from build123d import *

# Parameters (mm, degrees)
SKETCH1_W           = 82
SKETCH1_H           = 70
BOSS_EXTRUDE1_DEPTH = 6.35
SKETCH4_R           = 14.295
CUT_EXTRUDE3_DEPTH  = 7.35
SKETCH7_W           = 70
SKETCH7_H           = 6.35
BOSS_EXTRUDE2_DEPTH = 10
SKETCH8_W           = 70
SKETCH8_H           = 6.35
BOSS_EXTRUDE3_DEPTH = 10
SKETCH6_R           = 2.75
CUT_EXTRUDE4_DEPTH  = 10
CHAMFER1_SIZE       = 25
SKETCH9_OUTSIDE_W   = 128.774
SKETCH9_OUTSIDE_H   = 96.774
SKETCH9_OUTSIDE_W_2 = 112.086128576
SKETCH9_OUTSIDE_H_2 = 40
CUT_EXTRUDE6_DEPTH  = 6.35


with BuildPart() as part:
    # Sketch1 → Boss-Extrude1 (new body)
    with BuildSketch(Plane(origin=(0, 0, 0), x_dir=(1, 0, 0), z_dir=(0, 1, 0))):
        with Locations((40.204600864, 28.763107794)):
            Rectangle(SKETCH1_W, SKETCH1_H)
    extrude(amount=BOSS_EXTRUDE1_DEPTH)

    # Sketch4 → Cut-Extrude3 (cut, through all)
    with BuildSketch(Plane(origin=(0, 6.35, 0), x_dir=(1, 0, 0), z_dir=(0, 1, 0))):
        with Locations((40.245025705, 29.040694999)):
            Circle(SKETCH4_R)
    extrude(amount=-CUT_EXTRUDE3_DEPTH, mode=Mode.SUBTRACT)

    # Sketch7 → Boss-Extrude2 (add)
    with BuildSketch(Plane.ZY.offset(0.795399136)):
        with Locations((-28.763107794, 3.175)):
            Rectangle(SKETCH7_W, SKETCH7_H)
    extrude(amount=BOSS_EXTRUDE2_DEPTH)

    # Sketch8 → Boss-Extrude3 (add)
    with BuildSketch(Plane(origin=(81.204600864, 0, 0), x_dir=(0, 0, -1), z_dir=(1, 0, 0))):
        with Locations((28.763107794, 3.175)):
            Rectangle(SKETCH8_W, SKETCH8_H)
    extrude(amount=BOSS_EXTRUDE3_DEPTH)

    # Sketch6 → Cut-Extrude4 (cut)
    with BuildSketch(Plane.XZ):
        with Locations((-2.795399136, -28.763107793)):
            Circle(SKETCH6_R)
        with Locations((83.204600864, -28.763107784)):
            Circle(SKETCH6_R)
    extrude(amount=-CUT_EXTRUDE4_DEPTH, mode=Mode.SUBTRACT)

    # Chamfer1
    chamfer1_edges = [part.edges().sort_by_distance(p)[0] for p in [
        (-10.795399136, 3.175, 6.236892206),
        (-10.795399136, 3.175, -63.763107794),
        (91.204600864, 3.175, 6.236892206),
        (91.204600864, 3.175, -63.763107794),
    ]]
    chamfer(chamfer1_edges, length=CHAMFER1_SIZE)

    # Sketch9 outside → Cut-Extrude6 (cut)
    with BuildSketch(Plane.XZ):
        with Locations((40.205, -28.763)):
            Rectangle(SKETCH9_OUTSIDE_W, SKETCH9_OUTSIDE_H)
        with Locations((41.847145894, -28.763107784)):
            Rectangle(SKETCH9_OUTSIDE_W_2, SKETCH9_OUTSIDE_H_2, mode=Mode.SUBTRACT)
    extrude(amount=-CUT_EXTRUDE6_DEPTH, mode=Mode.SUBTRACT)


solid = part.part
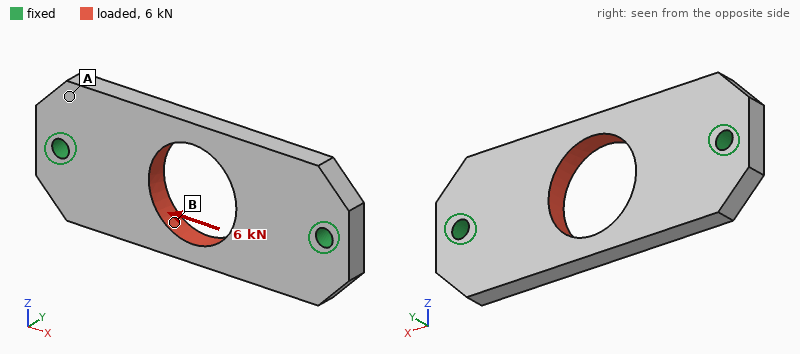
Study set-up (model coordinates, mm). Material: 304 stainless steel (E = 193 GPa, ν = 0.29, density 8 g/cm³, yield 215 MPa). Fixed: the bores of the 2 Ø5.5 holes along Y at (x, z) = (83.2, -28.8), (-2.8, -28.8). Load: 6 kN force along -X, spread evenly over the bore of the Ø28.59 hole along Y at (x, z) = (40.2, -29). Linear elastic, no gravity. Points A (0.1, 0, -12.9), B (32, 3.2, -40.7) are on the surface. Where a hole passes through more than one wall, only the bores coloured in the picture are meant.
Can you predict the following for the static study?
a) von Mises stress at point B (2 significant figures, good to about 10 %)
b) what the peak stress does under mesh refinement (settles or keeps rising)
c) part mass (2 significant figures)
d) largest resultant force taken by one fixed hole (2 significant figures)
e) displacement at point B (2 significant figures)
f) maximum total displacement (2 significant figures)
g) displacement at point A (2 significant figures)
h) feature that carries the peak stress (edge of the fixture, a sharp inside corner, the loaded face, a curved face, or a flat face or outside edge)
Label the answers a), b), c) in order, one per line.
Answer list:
a) 21 MPa
b) keeps rising
c) 160 g
d) 3.0 kN
e) 3.7 µm
f) 4.1 µm
g) 1.9 µm
h) edge of the fixture
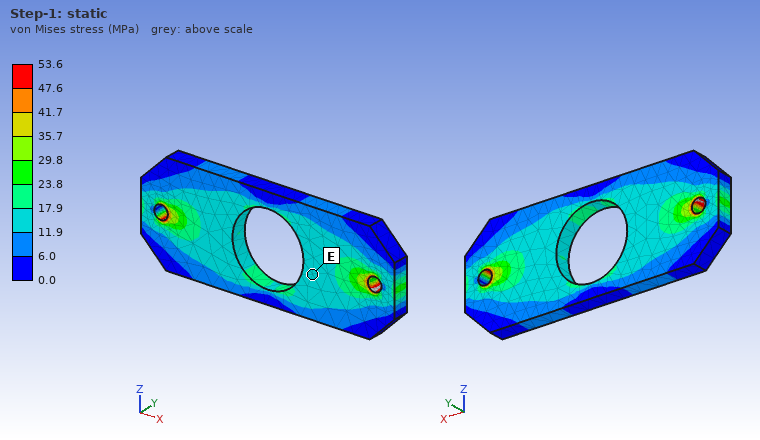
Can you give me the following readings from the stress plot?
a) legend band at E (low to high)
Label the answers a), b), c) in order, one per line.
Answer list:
a) 11.9 to 17.9 MPa
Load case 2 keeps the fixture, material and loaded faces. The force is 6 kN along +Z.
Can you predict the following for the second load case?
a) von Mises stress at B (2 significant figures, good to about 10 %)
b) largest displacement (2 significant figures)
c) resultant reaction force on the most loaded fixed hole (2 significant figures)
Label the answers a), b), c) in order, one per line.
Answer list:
a) 44 MPa
b) 19 µm
c) 3.0 kN
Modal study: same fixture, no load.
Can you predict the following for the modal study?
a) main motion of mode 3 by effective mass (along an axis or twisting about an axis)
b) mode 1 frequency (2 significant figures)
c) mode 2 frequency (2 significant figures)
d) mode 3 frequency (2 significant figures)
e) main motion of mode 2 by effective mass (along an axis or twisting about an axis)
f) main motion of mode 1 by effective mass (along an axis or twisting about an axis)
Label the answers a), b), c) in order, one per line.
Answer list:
a) twisting about Z
b) 4100 Hz
c) 5000 Hz
d) 8800 Hz
e) twisting about X
f) along Y
